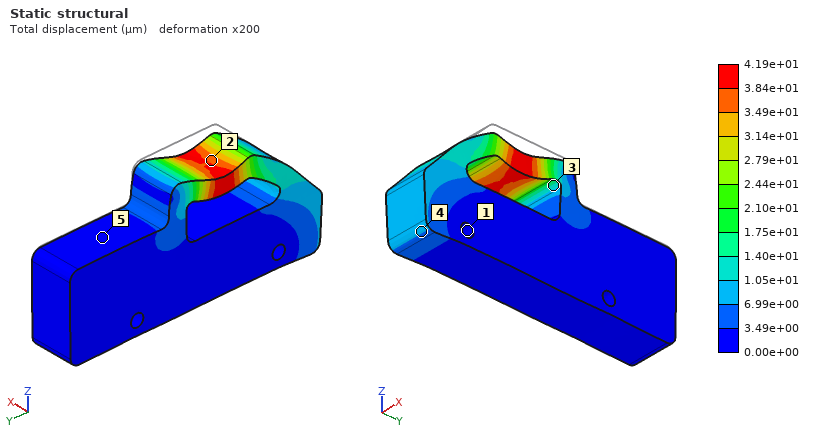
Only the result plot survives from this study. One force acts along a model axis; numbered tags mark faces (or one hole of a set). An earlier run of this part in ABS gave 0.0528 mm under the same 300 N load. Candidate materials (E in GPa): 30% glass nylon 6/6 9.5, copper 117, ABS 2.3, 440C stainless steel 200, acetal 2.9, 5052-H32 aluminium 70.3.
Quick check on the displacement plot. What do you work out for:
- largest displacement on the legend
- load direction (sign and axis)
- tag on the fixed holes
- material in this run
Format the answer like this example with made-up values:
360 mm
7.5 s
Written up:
4.19e+01 µm
-Z
1
acetal
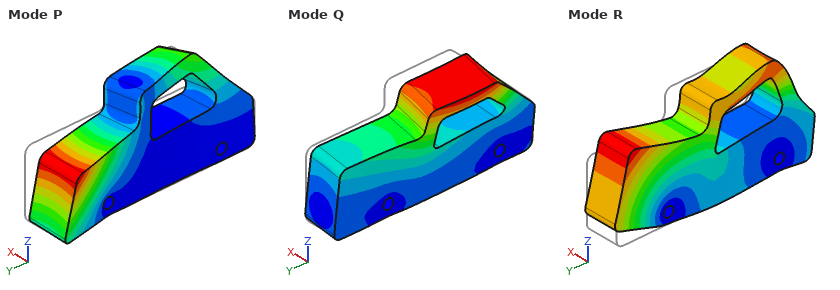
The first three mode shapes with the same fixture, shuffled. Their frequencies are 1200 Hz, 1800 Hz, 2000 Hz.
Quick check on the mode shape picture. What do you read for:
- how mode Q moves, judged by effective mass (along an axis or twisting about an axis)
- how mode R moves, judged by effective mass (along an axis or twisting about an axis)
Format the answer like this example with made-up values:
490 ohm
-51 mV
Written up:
along X
along Y
